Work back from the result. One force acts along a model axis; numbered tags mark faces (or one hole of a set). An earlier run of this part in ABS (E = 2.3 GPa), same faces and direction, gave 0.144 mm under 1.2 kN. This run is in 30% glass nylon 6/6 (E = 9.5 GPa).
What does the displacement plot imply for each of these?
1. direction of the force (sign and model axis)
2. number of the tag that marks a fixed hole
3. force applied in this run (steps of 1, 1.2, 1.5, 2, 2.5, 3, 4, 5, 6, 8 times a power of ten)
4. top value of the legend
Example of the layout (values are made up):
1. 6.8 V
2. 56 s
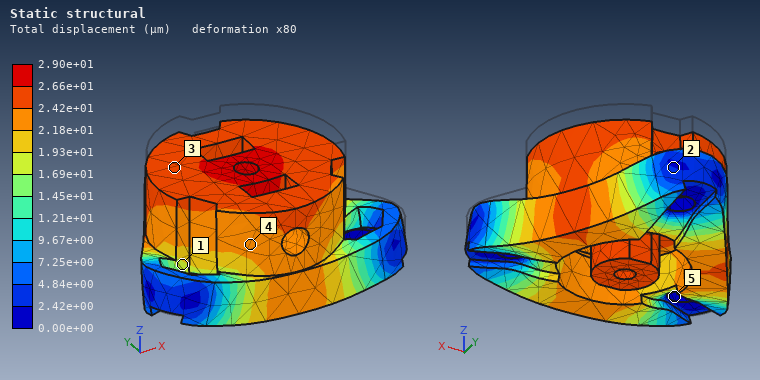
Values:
1. -Z
2. 5
3. 1 kN
4. 2.90e+01 µm
